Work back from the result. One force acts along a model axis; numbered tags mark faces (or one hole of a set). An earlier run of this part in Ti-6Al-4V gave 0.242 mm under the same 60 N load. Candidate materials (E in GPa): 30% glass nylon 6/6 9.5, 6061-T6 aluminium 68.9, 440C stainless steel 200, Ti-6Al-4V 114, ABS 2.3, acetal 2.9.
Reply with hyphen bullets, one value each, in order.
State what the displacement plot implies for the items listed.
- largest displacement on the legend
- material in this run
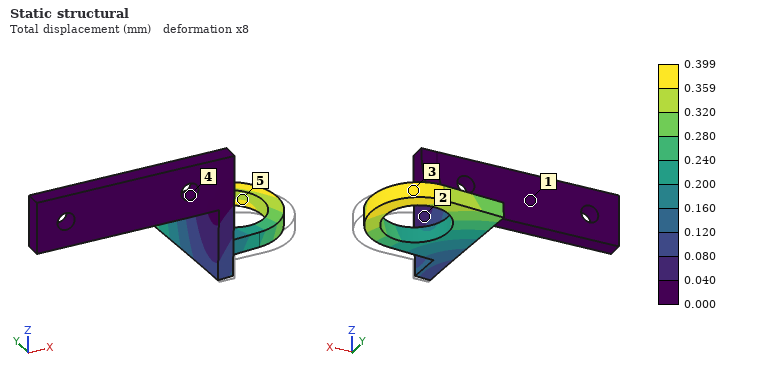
- 0.399 mm
- 6061-T6 aluminium
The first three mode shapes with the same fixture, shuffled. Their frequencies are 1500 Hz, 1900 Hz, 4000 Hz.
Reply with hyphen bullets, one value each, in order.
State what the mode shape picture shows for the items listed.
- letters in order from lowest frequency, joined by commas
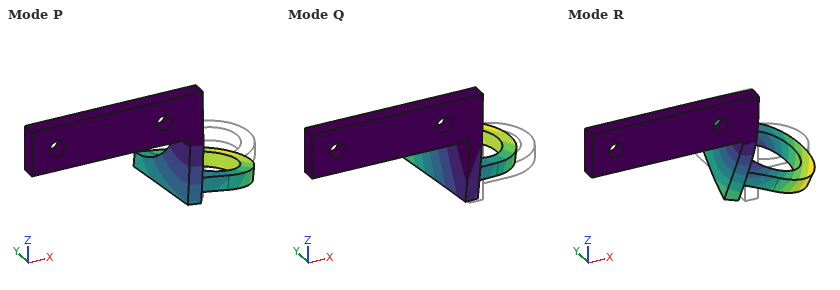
- Q, P, R
